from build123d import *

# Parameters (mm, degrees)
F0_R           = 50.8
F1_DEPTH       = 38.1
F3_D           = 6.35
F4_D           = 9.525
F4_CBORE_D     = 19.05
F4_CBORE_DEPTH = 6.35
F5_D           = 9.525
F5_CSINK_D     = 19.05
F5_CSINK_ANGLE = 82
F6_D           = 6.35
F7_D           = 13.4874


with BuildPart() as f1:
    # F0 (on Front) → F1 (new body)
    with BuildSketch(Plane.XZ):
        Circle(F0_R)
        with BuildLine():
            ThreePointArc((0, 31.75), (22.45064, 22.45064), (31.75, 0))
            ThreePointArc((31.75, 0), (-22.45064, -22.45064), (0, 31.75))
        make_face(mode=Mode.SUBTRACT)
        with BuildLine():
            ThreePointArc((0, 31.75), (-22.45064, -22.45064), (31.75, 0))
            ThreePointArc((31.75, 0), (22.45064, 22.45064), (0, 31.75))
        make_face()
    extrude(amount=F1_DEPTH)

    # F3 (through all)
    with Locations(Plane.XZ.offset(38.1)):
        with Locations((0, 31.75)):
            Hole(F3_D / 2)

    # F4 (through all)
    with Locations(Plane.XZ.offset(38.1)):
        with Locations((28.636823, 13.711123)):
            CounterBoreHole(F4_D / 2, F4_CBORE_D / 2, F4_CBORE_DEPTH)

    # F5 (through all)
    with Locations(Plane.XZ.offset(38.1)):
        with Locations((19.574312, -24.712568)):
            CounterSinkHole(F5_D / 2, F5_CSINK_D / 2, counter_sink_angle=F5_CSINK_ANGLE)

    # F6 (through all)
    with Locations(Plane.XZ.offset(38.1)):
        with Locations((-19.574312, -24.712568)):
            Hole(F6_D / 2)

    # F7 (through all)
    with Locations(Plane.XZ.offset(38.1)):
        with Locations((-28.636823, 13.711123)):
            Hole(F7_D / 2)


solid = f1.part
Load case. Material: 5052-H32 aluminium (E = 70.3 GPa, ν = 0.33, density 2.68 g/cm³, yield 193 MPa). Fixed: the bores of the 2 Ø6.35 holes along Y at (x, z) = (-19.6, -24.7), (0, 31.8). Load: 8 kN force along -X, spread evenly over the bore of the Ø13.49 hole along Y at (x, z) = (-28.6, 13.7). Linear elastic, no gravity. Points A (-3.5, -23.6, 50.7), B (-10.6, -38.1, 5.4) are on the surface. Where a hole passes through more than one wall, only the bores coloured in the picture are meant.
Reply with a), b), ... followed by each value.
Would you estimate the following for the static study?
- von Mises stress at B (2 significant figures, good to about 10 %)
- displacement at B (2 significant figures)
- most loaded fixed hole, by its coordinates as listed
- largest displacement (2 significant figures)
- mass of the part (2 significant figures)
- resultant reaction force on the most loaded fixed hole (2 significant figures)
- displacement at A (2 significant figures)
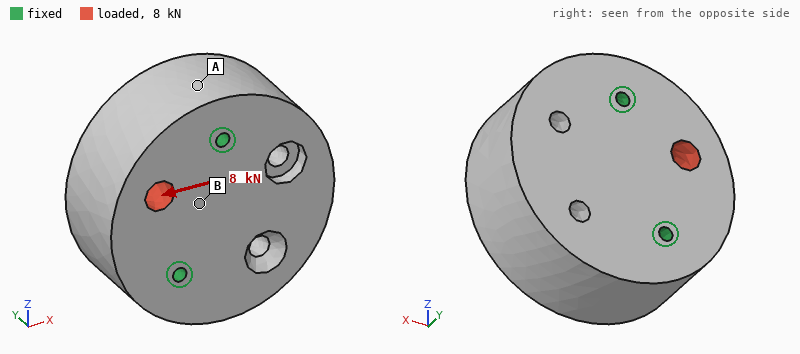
a) 3.0 MPa
b) 1.9 µm
c) (0, 31.8)
d) 3.9 µm
e) 790 g
f) 5.6 kN
g) 0.94 µm
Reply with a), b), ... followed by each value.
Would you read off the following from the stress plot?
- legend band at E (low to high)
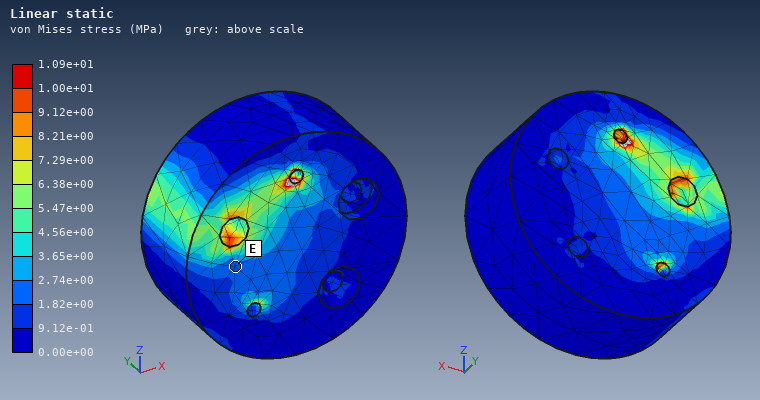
a) 1.82e+00 to 2.74e+00 MPa
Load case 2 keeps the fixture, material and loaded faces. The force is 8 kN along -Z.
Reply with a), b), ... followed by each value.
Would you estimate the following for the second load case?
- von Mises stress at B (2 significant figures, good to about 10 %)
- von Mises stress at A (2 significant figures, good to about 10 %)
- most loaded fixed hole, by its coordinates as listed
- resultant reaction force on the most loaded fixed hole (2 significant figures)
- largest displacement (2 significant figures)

a) 3.3 MPa
b) 2.5 MPa
c) (-19.6, -24.7)
d) 5.4 kN
e) 4.2 µm
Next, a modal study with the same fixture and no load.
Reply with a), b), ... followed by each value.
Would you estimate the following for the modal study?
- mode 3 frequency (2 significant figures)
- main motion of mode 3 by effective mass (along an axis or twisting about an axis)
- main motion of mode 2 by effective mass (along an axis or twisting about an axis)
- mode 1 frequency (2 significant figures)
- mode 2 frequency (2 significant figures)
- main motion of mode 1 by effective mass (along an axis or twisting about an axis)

a) 12 kHz
b) along Y
c) along Z
d) 6300 Hz
e) 10 kHz
f) along Y
